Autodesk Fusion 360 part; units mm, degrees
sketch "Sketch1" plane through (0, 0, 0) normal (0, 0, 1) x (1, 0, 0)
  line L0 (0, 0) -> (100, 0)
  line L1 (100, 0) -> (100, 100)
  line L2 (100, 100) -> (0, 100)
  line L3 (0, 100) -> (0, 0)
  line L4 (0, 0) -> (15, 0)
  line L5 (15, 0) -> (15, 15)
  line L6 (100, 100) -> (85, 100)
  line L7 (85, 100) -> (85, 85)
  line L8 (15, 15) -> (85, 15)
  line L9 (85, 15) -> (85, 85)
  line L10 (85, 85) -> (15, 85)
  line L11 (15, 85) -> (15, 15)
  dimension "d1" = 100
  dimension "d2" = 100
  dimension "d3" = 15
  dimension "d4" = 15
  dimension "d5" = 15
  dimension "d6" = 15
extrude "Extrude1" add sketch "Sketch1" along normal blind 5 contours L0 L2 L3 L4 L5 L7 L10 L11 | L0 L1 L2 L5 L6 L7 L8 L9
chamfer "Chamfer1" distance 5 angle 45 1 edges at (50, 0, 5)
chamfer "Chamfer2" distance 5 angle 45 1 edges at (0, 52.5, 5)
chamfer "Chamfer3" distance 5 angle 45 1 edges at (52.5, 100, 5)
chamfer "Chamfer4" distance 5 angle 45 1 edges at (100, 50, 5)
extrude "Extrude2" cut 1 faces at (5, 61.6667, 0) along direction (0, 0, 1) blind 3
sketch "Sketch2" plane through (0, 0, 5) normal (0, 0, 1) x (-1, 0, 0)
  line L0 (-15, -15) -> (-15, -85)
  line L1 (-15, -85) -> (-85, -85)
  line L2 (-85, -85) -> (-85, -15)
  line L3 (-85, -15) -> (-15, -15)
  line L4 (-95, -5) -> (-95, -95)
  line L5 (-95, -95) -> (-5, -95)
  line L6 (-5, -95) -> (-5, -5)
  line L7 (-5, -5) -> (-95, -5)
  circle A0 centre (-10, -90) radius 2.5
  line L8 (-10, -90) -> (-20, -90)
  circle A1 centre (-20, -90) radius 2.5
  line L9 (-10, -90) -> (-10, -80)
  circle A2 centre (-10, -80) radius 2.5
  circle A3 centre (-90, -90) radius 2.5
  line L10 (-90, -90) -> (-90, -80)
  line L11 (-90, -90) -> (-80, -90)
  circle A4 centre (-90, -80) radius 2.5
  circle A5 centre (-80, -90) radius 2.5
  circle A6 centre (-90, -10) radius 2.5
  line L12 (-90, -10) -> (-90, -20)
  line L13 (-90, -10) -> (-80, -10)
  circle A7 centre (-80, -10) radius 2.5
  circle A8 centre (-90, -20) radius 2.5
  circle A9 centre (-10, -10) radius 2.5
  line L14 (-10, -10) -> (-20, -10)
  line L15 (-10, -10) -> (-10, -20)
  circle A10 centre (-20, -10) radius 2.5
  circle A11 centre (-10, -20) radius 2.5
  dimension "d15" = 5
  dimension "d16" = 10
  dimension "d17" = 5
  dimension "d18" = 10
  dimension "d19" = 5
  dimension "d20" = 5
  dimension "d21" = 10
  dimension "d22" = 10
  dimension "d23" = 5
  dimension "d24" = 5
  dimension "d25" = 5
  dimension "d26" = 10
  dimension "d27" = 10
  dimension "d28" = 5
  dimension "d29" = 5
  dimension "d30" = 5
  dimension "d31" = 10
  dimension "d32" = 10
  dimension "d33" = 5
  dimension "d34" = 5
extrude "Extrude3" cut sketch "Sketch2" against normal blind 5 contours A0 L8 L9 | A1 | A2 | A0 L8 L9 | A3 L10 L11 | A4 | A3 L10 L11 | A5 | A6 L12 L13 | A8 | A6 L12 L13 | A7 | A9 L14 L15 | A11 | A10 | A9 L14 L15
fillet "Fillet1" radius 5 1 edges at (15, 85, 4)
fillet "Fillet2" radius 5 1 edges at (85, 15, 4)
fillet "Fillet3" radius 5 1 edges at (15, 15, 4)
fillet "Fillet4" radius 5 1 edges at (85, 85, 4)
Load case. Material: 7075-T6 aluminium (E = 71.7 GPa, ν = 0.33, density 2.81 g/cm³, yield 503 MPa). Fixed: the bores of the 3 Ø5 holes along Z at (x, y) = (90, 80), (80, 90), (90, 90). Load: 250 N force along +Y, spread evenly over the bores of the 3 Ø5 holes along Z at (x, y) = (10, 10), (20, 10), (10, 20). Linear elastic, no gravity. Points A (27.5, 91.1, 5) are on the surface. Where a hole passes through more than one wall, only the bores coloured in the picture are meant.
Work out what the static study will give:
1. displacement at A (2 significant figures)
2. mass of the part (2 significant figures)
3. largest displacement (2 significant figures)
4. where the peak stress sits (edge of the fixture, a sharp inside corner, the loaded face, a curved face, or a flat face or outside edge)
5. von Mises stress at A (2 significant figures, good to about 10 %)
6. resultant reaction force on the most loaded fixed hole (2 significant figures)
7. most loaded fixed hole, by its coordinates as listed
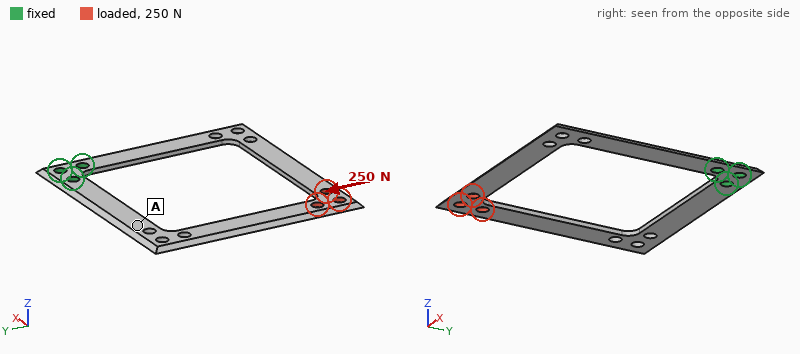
0.67 mm
19 g
1.2 mm
edge of the fixture
24 MPa
480 N
(80, 90)
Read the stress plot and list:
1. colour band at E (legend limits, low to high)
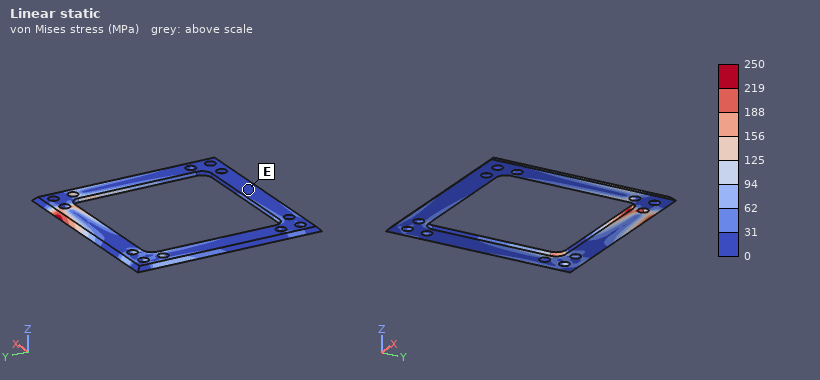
0 to 31 MPa
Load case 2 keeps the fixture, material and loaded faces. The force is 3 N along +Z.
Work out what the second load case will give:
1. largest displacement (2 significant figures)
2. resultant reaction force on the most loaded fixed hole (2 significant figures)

1.6 mm
2.1 N
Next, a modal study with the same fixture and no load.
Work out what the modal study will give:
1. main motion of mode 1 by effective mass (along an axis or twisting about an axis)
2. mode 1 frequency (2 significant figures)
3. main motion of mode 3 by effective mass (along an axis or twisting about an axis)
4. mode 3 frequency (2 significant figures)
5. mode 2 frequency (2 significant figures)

along Z
110 Hz
along Z
430 Hz
230 Hz
